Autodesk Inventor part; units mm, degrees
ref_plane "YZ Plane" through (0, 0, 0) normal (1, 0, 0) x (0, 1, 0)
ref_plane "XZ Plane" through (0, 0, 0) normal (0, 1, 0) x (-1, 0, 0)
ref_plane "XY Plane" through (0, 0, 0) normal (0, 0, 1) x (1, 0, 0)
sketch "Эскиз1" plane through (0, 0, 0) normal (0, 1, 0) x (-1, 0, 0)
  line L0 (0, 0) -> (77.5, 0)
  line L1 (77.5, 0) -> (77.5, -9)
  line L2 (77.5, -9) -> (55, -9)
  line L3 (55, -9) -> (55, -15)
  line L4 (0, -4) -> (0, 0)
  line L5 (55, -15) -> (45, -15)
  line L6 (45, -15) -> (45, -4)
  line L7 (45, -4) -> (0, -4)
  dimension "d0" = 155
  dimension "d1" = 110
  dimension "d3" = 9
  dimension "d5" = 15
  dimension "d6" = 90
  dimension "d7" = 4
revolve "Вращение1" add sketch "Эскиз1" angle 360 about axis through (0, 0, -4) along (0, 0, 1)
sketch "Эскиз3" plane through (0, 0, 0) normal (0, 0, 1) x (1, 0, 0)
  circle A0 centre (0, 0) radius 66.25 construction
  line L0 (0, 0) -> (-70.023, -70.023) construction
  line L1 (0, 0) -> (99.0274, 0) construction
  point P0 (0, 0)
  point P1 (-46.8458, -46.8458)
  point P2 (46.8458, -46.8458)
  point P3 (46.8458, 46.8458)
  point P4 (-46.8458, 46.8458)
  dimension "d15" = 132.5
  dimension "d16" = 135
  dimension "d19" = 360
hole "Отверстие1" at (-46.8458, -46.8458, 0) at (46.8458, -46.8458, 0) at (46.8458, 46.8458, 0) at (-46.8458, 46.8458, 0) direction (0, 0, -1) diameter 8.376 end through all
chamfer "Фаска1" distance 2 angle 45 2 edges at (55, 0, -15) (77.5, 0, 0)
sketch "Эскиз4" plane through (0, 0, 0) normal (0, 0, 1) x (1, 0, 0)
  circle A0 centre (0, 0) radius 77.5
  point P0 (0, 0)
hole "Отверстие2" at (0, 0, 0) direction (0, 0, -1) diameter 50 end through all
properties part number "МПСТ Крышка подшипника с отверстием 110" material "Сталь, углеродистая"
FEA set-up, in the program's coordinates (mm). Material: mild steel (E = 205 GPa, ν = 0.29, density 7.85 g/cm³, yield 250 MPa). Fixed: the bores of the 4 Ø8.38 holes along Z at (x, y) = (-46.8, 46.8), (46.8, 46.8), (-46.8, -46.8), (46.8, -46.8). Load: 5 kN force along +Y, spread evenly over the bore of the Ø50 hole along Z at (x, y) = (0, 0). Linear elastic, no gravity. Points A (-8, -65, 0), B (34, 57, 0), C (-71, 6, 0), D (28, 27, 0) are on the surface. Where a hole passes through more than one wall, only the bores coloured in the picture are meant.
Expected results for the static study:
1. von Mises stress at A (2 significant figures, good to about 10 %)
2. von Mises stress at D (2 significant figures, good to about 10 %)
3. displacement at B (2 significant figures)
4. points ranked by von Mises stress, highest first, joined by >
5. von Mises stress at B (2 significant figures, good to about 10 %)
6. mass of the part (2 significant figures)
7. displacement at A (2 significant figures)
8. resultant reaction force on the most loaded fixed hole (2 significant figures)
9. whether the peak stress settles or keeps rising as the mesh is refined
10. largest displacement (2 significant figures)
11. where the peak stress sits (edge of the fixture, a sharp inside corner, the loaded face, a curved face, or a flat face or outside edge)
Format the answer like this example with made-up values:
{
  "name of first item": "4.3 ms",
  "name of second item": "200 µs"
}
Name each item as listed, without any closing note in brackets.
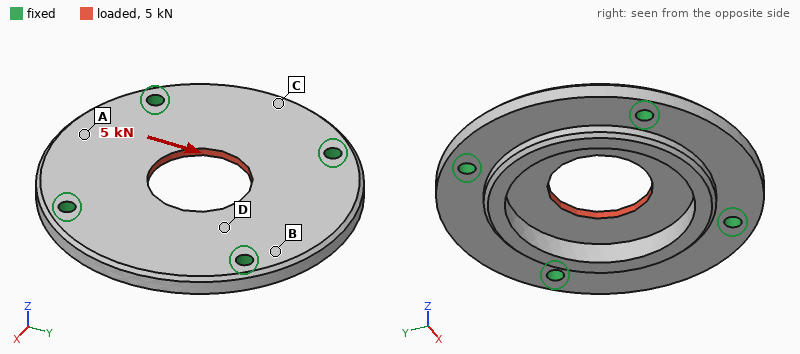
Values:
{
  "von Mises stress at A": "2.7 MPa",
  "von Mises stress at D": "6.9 MPa",
  "displacement at B": "0.71 µm",
  "points ranked by von Mises stress, highest first, joined by >": "D > B > A > C",
  "von Mises stress at B": "4.9 MPa",
  "mass of the part": "1.1 kg",
  "displacement at A": "1.6 µm",
  "resultant reaction force on the most loaded fixed hole": "1.3 kN",
  "whether the peak stress settles or keeps rising as the mesh is refined": "keeps rising",
  "largest displacement": "3.0 µm",
  "where the peak stress sits": "edge of the fixture"
}
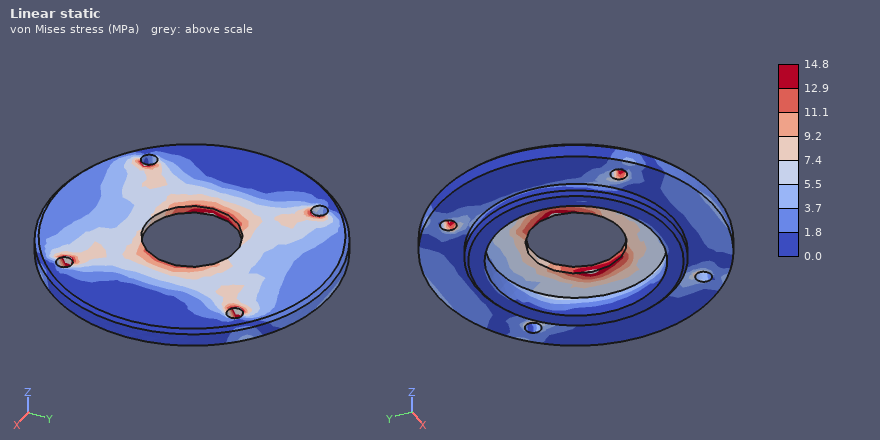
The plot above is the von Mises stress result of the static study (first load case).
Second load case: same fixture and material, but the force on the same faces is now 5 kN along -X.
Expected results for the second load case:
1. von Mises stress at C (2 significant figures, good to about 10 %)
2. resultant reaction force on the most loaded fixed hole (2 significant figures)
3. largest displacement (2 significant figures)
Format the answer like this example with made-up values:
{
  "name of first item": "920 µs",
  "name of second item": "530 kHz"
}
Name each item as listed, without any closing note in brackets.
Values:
{
  "von Mises stress at C": "2.7 MPa",
  "resultant reaction force on the most loaded fixed hole": "1.3 kN",
  "largest displacement": "2.9 µm"
}
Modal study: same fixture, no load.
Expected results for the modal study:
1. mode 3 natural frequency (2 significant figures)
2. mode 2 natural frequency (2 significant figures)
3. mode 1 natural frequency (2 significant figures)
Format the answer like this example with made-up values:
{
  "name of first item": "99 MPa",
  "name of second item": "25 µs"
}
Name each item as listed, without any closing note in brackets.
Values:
{
  "mode 3 natural frequency": "4900 Hz",
  "mode 2 natural frequency": "4900 Hz",
  "mode 1 natural frequency": "4300 Hz"
}
